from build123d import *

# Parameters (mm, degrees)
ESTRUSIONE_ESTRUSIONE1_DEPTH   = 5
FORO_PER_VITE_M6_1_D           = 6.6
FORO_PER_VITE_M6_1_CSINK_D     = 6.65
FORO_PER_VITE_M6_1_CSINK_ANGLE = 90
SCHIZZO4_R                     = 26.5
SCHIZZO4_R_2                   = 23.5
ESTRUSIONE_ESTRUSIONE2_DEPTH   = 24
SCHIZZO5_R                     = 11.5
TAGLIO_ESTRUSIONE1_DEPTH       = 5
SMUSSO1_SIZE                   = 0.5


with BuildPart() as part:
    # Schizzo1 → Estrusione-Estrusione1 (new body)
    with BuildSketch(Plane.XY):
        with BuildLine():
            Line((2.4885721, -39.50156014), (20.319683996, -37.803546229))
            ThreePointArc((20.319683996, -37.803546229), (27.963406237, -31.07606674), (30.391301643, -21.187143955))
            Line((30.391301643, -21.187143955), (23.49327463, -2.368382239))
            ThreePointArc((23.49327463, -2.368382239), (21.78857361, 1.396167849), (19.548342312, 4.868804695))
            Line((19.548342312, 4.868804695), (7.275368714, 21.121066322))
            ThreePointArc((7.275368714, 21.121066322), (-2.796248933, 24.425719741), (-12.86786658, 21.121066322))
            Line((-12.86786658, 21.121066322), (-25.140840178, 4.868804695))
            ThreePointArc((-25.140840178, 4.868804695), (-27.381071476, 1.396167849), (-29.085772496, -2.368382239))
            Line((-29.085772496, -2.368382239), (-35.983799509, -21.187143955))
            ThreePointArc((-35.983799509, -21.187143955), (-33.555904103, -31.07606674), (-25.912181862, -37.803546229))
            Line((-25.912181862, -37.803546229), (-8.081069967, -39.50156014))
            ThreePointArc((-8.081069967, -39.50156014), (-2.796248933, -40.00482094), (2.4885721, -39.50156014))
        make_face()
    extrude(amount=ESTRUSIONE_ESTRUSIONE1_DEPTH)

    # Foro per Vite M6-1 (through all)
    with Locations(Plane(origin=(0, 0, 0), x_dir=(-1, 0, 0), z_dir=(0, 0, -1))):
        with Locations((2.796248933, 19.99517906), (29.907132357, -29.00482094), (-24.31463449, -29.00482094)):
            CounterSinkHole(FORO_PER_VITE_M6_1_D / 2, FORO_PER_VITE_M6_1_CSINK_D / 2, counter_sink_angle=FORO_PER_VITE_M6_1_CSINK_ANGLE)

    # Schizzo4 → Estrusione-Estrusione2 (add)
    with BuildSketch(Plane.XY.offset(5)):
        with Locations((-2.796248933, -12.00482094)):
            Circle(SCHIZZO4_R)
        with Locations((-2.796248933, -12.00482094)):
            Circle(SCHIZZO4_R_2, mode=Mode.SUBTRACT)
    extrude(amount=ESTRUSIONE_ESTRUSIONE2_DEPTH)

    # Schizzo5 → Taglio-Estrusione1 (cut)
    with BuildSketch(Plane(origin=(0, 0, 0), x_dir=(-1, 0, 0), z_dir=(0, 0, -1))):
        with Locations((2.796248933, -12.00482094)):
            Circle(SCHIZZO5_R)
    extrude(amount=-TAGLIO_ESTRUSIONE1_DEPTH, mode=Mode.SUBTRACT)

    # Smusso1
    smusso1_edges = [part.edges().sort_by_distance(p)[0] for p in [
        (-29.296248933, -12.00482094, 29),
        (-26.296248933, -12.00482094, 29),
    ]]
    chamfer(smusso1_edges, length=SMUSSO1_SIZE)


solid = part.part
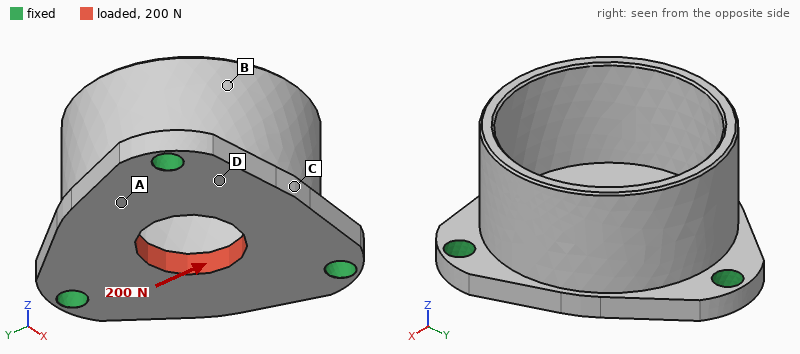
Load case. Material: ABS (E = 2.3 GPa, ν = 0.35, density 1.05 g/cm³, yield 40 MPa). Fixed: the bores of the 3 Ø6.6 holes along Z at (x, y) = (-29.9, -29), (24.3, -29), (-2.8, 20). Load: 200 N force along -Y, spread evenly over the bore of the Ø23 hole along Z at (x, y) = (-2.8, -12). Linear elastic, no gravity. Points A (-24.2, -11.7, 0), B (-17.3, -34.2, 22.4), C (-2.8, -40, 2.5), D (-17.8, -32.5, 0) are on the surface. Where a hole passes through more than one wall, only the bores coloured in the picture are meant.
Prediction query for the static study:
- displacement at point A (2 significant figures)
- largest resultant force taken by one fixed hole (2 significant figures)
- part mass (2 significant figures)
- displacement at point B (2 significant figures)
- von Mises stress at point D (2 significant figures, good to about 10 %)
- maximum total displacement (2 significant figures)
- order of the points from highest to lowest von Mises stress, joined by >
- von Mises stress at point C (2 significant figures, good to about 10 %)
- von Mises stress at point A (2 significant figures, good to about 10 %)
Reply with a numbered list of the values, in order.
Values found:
1. 8.1 µm
2. 69 N
3. 25 g
4. 8.3 µm
5. 0.62 MPa
6. 18 µm
7. C > D > A > B
8. 0.87 MPa
9. 0.41 MPa
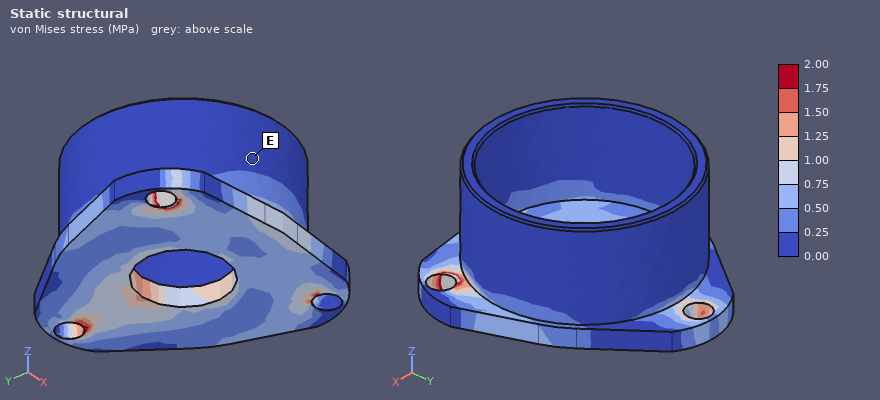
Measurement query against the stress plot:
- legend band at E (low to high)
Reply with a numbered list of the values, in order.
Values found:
1. 0.00 to 0.25 MPa
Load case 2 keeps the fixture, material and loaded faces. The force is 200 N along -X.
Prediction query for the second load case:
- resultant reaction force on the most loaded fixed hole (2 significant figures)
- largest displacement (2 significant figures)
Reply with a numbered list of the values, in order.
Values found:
1. 67 N
2. 17 µm
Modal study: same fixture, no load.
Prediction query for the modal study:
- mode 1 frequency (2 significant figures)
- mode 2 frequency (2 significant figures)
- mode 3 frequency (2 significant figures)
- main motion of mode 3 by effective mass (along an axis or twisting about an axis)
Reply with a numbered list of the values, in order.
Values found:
1. 1700 Hz
2. 1700 Hz
3. 2800 Hz
4. along Z
